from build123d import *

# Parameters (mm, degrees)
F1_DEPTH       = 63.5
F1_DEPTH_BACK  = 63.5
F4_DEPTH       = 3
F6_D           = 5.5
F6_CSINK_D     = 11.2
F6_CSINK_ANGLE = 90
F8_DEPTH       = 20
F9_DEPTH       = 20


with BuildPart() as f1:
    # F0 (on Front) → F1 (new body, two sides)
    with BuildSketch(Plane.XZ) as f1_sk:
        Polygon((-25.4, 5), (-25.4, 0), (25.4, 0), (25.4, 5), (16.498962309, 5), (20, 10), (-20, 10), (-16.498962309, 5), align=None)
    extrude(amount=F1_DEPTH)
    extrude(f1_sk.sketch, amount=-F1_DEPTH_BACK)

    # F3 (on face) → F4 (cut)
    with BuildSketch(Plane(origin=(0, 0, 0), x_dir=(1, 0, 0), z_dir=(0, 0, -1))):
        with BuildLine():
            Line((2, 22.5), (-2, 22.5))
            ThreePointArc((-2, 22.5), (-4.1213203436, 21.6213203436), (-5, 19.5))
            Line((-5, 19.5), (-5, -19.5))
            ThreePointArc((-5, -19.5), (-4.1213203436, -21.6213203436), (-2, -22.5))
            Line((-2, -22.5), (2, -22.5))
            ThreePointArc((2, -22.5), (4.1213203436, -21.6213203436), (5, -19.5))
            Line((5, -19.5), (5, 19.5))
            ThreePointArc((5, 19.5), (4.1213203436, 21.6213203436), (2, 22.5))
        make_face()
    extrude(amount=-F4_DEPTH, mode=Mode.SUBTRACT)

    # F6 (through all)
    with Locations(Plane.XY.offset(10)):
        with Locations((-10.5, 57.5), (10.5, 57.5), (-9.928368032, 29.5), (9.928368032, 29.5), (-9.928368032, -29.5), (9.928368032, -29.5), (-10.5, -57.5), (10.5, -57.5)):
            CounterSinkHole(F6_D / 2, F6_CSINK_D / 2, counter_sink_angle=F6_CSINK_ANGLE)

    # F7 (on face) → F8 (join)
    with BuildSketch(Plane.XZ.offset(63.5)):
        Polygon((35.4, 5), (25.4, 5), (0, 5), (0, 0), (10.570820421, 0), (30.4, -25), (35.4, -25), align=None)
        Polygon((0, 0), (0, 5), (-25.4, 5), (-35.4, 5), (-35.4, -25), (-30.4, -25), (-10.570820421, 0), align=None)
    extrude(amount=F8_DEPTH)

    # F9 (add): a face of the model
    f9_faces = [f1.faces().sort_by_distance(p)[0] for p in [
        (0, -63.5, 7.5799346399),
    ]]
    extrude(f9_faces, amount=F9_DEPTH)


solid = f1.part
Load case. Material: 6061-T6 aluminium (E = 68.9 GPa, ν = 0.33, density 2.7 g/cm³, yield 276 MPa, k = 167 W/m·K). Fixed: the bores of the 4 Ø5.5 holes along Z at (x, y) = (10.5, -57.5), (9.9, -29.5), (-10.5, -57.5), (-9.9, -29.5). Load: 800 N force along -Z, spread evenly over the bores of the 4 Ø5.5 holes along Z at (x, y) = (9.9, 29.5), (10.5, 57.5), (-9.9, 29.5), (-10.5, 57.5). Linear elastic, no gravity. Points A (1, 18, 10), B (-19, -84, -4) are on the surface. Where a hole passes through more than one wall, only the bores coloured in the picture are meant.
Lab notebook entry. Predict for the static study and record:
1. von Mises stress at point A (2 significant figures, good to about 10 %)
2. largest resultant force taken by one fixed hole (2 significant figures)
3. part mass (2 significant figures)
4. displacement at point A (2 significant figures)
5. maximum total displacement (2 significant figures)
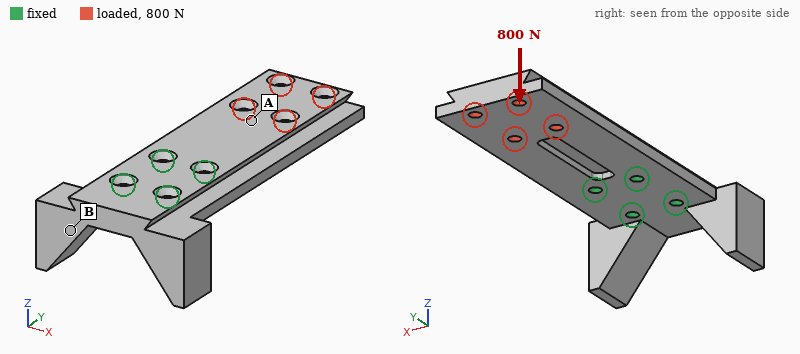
33 MPa
770 N
210 g
0.27 mm
0.73 mm
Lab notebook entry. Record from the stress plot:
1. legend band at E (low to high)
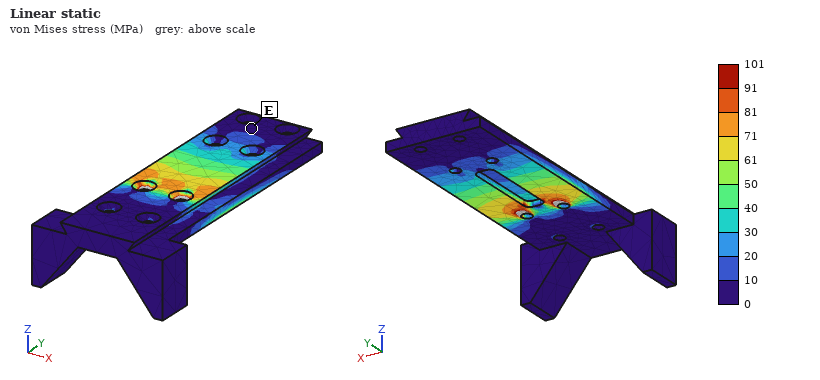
0 to 10 MPa
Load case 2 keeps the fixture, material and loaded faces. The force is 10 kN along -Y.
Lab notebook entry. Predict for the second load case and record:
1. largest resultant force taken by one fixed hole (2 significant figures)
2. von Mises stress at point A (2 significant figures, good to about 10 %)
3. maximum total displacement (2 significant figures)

4.3 kN
8.1 MPa
0.23 mm
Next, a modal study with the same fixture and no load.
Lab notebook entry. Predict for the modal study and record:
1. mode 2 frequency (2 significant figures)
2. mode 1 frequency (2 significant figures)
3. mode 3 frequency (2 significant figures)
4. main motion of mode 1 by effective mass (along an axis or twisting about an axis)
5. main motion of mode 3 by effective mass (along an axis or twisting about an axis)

2800 Hz
880 Hz
3400 Hz
along Z
along X
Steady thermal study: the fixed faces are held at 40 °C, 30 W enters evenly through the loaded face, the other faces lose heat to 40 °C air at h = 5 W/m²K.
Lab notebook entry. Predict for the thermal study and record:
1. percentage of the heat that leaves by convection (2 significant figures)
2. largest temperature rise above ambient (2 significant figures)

4.2 %
33 K
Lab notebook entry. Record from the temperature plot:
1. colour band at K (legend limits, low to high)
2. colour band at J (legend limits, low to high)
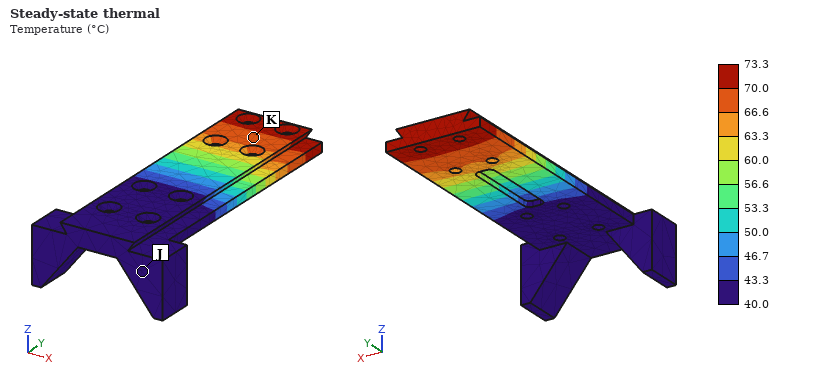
66.6 to 70.0 °C
40.0 to 43.3 °C
